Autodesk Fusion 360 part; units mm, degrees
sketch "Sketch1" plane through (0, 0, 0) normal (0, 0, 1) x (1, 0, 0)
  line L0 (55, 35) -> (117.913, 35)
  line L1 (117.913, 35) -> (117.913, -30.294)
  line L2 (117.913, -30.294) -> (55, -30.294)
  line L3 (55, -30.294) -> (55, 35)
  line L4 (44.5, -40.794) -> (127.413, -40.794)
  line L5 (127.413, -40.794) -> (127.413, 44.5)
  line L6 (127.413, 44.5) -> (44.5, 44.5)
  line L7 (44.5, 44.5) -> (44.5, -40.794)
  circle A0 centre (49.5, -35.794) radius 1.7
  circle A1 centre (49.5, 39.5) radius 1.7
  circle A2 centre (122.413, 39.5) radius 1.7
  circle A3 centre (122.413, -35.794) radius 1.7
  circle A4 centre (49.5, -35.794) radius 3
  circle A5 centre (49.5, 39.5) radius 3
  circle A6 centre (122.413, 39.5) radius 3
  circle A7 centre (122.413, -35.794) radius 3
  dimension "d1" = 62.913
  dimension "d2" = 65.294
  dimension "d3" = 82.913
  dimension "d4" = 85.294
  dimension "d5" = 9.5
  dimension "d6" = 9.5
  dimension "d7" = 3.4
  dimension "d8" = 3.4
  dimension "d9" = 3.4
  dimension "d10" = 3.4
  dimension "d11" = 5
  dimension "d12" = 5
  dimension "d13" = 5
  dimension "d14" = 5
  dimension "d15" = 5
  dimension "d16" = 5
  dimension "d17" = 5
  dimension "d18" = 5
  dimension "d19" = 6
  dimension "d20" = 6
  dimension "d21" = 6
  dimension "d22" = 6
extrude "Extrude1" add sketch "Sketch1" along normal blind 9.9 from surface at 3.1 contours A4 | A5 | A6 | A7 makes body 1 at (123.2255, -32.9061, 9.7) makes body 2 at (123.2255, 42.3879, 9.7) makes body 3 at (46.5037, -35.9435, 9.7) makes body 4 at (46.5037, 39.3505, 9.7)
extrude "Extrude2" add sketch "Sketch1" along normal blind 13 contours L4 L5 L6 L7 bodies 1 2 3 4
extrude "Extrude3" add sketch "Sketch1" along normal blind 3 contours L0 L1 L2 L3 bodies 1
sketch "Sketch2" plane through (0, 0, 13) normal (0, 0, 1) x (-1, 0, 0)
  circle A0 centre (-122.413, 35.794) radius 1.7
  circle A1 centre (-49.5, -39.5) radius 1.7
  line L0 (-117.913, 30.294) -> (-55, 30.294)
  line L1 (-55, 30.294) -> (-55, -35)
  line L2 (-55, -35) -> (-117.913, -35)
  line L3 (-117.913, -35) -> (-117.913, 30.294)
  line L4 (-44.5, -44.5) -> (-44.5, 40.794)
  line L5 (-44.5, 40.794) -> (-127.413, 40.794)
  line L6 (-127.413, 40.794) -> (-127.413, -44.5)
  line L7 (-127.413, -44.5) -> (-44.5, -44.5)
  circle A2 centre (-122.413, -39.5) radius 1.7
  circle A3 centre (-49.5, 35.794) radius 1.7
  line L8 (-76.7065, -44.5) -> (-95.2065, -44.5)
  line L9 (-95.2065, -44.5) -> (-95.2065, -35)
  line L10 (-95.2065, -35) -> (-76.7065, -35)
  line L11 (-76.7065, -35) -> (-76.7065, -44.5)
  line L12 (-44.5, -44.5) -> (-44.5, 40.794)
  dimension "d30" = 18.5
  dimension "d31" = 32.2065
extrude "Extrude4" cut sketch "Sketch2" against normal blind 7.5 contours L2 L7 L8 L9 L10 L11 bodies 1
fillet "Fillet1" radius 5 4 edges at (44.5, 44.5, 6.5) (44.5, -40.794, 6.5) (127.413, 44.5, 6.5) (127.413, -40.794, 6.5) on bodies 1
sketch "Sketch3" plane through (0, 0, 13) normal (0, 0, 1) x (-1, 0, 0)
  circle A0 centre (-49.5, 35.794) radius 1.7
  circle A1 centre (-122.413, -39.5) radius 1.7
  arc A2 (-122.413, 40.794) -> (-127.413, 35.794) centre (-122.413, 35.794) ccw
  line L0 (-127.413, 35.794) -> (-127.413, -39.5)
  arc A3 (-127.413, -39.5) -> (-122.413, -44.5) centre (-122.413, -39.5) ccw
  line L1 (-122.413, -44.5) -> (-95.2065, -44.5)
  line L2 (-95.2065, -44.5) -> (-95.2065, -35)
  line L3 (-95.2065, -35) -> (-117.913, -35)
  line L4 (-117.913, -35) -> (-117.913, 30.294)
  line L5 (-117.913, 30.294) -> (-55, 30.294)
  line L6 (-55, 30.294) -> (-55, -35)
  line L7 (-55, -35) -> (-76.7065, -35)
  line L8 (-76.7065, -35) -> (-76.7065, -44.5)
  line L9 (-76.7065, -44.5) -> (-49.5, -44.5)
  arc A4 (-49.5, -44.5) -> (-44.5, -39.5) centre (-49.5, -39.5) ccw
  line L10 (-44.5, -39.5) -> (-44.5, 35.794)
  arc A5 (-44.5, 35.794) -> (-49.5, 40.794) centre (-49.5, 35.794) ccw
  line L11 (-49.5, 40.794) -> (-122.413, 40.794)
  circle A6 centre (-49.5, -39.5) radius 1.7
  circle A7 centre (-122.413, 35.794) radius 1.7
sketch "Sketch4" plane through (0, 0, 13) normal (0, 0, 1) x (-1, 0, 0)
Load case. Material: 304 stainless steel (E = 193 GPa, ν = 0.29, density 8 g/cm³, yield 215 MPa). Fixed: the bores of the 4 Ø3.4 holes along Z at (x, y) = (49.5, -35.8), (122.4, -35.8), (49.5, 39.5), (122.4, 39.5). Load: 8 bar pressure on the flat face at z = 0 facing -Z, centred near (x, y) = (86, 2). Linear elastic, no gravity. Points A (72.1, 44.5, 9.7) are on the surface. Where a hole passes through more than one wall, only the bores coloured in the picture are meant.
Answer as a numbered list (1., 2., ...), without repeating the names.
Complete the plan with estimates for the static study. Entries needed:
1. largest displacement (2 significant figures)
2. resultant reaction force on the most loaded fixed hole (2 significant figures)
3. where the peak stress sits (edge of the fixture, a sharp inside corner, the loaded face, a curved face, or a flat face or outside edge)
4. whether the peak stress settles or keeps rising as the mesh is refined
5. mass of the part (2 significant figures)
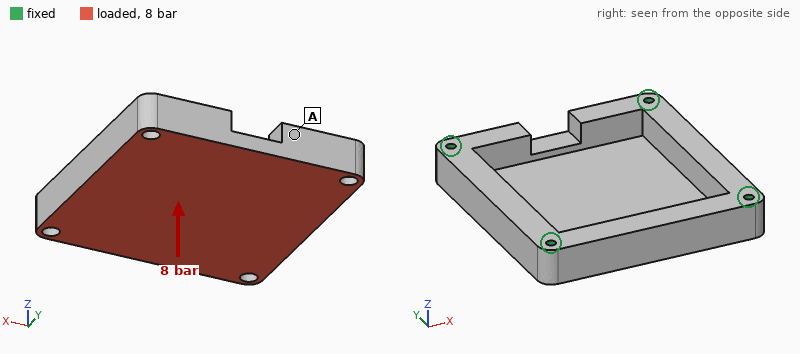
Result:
1. 64 µm
2. 2.1 kN
3. edge of the fixture
4. keeps rising
5. 390 g
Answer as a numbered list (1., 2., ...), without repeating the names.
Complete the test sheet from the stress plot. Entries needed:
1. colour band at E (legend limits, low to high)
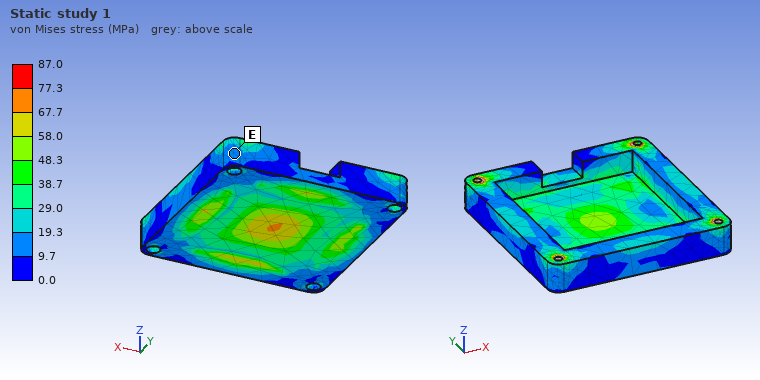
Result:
1. 9.7 to 19.3 MPa
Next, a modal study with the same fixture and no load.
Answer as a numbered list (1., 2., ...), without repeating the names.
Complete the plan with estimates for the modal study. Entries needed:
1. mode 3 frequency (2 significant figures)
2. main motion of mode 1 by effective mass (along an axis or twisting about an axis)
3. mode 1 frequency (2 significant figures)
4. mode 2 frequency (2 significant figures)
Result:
1. 7900 Hz
2. along Z
3. 4600 Hz
4. 7700 Hz
